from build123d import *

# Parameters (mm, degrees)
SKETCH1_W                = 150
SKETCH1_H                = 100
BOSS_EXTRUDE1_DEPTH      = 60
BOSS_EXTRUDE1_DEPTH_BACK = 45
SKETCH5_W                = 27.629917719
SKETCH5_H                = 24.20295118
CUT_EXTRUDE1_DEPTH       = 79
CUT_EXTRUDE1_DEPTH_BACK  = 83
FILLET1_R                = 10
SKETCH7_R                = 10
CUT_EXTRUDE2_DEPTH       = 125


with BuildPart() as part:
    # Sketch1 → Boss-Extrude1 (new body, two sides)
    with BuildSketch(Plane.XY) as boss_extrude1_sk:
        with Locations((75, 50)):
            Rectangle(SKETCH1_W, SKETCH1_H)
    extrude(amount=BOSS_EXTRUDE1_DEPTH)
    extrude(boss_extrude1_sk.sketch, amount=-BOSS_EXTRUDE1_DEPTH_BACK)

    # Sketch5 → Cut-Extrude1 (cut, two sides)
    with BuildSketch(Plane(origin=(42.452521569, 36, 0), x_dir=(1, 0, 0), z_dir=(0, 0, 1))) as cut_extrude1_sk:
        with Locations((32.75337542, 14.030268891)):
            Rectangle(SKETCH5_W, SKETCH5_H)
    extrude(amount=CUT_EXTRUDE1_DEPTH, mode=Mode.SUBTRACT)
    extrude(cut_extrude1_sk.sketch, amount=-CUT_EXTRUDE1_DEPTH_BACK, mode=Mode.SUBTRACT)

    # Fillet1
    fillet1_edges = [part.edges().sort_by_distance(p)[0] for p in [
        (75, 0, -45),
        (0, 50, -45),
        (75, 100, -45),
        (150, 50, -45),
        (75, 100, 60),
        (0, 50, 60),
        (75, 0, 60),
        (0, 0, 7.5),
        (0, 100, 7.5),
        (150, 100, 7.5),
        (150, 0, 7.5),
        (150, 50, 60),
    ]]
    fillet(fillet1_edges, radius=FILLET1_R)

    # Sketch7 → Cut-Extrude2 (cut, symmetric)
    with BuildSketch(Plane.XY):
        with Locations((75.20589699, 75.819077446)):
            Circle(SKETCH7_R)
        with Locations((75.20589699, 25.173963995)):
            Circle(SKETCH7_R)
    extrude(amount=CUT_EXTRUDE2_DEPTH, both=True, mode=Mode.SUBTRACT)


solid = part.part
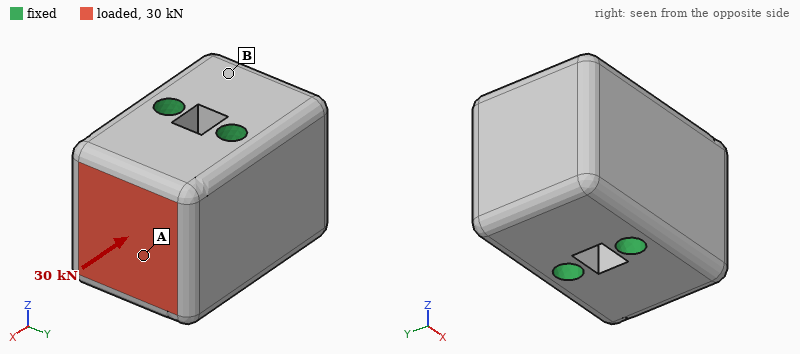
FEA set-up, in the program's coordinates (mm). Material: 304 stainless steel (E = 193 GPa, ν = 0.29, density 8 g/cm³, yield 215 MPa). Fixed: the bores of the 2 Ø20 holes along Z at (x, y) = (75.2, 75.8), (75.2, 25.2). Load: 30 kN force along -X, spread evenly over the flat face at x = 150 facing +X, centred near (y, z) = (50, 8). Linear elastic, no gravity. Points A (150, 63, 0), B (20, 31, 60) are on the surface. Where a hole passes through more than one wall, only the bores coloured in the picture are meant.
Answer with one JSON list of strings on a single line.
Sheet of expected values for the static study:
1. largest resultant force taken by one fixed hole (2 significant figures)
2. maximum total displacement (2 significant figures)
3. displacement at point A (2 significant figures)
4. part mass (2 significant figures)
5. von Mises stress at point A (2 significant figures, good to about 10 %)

["15 kN", "1.5 µm", "1.5 µm", "11 kg", "2.7 MPa"]
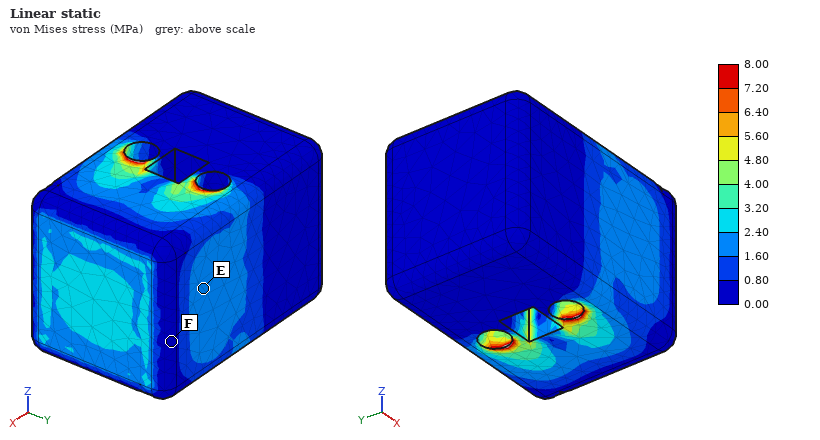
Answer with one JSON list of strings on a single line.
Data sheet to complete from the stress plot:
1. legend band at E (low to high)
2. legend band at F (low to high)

["1.60 to 2.40 MPa", "0.00 to 0.80 MPa"]
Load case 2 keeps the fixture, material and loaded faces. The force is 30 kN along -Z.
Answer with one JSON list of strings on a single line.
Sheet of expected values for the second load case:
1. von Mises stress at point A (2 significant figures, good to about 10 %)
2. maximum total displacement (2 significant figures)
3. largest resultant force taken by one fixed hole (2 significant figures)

["7.8 MPa", "6.3 µm", "15 kN"]
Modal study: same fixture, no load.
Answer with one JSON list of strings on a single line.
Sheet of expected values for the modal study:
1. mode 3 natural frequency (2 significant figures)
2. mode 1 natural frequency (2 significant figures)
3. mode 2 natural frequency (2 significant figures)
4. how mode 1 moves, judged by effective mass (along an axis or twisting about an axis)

["8100 Hz", "7100 Hz", "8000 Hz", "twisting about Z"]
